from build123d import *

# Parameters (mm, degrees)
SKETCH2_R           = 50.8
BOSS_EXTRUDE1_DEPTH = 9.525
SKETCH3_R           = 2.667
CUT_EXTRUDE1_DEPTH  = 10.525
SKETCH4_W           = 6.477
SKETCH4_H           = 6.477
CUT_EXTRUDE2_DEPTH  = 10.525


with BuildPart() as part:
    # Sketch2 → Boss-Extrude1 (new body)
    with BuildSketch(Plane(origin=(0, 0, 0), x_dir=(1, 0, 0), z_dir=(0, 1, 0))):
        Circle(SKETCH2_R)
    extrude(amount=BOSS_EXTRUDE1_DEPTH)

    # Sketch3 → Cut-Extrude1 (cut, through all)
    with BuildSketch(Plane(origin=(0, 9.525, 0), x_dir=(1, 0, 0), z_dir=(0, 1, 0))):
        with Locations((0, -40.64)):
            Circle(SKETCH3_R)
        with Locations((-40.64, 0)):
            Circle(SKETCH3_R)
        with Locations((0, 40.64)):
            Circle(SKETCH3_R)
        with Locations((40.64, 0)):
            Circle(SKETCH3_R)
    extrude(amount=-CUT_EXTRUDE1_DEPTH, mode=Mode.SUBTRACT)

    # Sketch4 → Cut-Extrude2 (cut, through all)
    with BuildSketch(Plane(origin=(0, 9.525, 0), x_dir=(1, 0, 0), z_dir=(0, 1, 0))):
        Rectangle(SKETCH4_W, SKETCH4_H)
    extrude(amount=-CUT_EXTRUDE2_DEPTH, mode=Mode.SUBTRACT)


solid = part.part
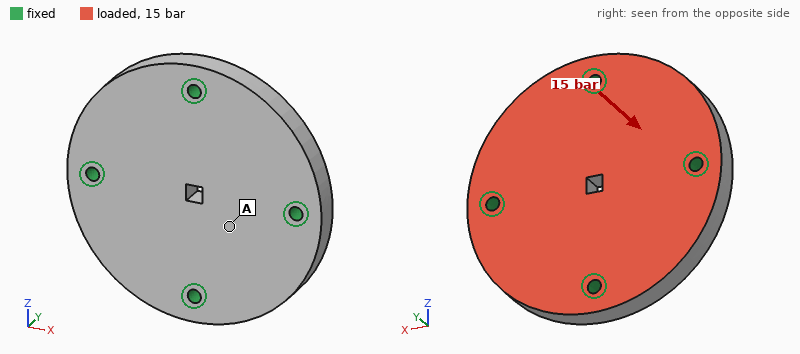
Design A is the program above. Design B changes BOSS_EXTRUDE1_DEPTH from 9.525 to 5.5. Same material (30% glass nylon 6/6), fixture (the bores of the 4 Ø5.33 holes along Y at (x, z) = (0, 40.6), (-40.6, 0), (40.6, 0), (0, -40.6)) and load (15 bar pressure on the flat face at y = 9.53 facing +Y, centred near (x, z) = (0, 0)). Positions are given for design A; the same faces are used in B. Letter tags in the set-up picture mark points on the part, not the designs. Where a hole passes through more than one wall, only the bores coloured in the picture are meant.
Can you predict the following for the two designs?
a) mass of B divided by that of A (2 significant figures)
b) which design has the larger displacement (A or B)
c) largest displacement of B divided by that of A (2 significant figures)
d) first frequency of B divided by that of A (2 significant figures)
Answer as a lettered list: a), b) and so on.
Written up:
a) 0.58
b) B
c) 4.0
d) 0.66
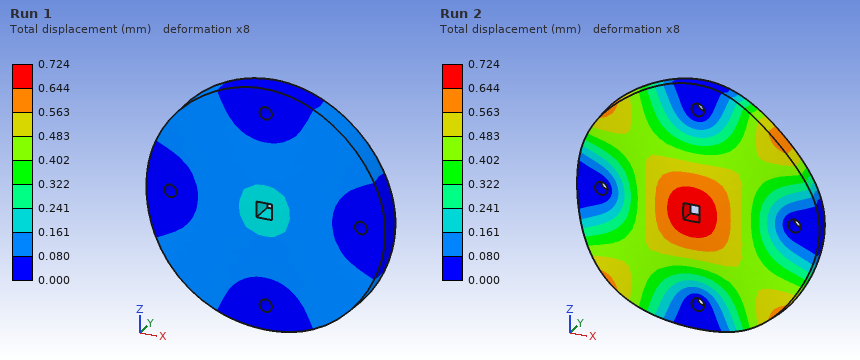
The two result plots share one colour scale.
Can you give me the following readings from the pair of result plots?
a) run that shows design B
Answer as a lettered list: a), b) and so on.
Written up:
a) Run 2
